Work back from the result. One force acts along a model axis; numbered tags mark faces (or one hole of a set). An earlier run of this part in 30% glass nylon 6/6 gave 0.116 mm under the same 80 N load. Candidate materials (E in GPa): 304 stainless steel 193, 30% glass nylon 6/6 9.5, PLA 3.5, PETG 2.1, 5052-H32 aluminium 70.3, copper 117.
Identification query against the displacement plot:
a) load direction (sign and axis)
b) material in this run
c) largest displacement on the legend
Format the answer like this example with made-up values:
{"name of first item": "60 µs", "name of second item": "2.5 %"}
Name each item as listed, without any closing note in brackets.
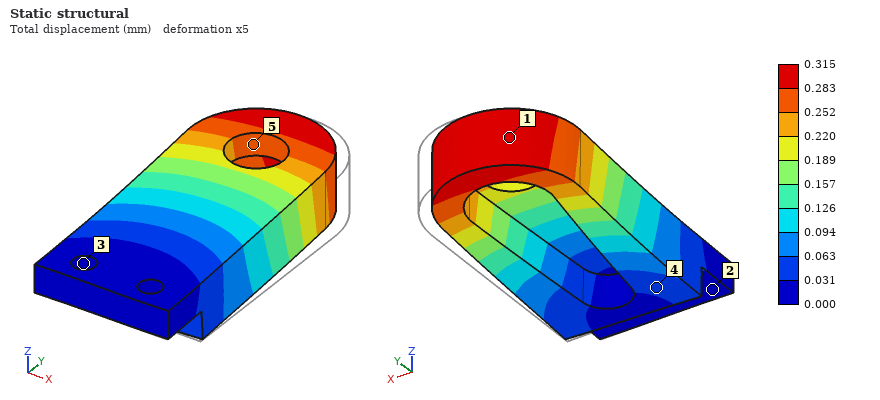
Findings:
{"load direction": "-X", "material in this run": "PLA", "largest displacement on the legend": "0.315 mm"}
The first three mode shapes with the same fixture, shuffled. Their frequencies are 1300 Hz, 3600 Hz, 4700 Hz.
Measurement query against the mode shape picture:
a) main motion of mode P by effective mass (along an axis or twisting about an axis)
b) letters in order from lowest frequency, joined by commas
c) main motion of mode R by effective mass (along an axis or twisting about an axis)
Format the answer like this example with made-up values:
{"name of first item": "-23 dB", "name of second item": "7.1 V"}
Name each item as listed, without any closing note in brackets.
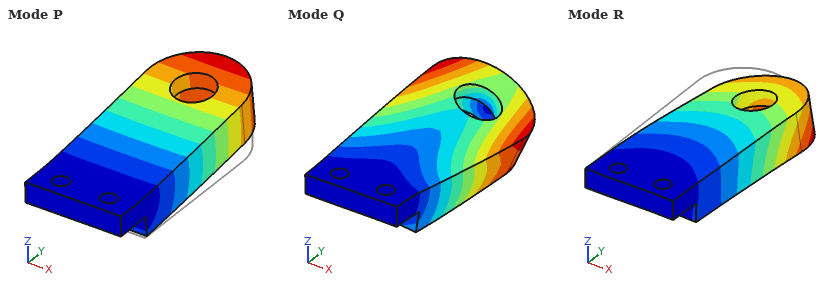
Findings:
{"main motion of mode P by effective mass": "along Z", "letters in order from lowest frequency, joined by commas": "P, R, Q", "main motion of mode R by effective mass": "along X"}
